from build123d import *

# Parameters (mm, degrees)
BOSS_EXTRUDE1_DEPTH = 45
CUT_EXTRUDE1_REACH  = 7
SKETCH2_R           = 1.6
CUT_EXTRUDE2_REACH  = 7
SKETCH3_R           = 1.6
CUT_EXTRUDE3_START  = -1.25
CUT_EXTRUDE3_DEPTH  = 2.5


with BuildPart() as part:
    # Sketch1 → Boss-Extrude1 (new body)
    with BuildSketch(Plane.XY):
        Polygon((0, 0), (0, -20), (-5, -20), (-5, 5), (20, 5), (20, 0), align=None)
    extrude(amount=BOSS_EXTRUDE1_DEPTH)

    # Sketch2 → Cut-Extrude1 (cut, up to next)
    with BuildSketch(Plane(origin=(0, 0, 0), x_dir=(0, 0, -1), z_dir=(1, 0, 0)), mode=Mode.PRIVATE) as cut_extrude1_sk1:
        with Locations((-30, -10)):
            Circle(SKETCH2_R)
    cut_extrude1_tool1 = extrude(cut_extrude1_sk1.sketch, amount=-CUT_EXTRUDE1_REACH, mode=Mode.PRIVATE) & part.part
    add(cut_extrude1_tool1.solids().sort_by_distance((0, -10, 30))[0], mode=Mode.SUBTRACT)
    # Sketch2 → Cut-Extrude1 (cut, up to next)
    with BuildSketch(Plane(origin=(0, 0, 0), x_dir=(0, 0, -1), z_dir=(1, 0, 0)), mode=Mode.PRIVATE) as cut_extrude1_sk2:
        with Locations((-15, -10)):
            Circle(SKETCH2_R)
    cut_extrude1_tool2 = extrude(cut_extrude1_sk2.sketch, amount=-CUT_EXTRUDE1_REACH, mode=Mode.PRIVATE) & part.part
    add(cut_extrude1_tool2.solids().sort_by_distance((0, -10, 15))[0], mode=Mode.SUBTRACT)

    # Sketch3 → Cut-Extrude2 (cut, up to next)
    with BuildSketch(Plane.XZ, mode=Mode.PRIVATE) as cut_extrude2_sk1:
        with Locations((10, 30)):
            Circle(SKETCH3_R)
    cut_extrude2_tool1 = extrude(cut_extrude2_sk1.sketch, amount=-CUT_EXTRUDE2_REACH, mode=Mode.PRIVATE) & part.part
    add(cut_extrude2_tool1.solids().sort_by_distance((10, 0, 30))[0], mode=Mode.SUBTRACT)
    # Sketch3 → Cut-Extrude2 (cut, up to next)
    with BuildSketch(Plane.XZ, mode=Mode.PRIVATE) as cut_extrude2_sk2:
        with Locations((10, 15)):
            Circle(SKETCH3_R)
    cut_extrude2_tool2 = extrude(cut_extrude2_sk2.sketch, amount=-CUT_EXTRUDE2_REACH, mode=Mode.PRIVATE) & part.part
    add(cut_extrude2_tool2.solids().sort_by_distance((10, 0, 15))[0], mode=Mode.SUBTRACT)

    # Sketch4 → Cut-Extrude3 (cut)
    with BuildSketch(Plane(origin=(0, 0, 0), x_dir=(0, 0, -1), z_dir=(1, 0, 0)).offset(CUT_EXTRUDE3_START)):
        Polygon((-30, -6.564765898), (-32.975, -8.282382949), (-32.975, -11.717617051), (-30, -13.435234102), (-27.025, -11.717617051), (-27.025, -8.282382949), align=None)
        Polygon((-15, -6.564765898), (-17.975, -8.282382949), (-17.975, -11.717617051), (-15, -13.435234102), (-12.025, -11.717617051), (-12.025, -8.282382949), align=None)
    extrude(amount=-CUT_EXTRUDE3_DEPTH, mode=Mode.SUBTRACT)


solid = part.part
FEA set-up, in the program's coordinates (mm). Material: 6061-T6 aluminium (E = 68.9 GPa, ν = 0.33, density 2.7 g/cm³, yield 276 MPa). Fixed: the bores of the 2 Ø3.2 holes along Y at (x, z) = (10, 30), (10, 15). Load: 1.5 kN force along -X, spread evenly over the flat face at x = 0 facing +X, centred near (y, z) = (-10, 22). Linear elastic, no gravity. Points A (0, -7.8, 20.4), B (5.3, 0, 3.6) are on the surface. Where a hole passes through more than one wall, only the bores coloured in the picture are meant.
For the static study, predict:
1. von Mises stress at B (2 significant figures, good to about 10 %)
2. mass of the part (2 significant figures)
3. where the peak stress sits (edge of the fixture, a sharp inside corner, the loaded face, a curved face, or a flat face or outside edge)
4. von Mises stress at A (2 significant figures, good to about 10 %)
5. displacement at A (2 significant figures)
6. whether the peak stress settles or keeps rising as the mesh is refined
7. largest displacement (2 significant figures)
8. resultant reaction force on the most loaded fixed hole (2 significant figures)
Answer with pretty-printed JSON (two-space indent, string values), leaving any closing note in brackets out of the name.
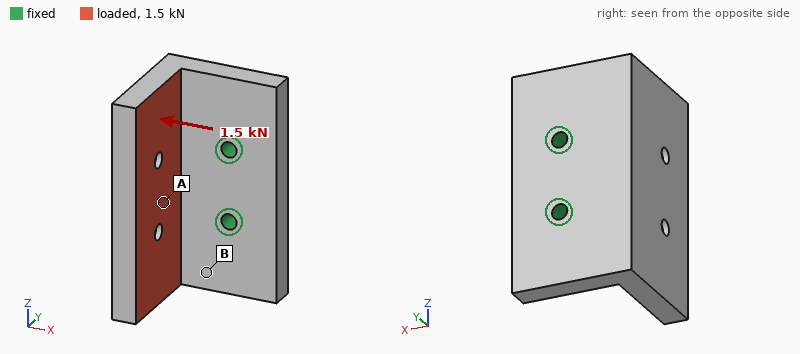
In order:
{
  "von Mises stress at B": "72 MPa",
  "mass of the part": "27 g",
  "where the peak stress sits": "edge of the fixture",
  "von Mises stress at A": "34 MPa",
  "displacement at A": "0.10 mm",
  "whether the peak stress settles or keeps rising as the mesh is refined": "keeps rising",
  "largest displacement": "0.25 mm",
  "resultant reaction force on the most loaded fixed hole": "750 N"
}
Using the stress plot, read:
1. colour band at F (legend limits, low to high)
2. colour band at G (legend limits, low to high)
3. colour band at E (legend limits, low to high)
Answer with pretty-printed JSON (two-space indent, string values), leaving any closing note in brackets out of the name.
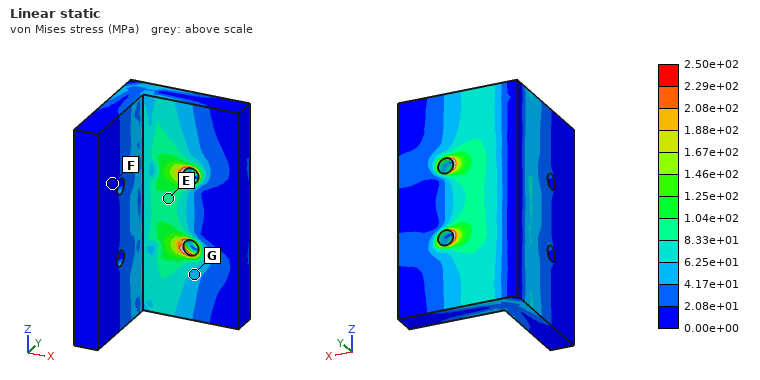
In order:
{
  "colour band at F": "0.00e+00 to 2.08e+01 MPa",
  "colour band at G": "4.17e+01 to 6.25e+01 MPa",
  "colour band at E": "8.33e+01 to 1.04e+02 MPa"
}
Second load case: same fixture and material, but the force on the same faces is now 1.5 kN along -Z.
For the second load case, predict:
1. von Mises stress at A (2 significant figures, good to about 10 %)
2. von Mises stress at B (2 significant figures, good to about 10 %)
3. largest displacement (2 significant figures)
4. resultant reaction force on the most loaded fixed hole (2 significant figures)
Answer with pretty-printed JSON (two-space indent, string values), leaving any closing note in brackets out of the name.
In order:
{
  "von Mises stress at A": "34 MPa",
  "von Mises stress at B": "28 MPa",
  "largest displacement": "99 µm",
  "resultant reaction force on the most loaded fixed hole": "1.4 kN"
}
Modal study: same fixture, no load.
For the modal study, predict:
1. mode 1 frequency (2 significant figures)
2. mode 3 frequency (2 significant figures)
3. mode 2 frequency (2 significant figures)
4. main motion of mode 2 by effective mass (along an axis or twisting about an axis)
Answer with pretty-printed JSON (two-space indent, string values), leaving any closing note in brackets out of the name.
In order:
{
  "mode 1 frequency": "4000 Hz",
  "mode 3 frequency": "9400 Hz",
  "mode 2 frequency": "5800 Hz",
  "main motion of mode 2 by effective mass": "along Z"
}
